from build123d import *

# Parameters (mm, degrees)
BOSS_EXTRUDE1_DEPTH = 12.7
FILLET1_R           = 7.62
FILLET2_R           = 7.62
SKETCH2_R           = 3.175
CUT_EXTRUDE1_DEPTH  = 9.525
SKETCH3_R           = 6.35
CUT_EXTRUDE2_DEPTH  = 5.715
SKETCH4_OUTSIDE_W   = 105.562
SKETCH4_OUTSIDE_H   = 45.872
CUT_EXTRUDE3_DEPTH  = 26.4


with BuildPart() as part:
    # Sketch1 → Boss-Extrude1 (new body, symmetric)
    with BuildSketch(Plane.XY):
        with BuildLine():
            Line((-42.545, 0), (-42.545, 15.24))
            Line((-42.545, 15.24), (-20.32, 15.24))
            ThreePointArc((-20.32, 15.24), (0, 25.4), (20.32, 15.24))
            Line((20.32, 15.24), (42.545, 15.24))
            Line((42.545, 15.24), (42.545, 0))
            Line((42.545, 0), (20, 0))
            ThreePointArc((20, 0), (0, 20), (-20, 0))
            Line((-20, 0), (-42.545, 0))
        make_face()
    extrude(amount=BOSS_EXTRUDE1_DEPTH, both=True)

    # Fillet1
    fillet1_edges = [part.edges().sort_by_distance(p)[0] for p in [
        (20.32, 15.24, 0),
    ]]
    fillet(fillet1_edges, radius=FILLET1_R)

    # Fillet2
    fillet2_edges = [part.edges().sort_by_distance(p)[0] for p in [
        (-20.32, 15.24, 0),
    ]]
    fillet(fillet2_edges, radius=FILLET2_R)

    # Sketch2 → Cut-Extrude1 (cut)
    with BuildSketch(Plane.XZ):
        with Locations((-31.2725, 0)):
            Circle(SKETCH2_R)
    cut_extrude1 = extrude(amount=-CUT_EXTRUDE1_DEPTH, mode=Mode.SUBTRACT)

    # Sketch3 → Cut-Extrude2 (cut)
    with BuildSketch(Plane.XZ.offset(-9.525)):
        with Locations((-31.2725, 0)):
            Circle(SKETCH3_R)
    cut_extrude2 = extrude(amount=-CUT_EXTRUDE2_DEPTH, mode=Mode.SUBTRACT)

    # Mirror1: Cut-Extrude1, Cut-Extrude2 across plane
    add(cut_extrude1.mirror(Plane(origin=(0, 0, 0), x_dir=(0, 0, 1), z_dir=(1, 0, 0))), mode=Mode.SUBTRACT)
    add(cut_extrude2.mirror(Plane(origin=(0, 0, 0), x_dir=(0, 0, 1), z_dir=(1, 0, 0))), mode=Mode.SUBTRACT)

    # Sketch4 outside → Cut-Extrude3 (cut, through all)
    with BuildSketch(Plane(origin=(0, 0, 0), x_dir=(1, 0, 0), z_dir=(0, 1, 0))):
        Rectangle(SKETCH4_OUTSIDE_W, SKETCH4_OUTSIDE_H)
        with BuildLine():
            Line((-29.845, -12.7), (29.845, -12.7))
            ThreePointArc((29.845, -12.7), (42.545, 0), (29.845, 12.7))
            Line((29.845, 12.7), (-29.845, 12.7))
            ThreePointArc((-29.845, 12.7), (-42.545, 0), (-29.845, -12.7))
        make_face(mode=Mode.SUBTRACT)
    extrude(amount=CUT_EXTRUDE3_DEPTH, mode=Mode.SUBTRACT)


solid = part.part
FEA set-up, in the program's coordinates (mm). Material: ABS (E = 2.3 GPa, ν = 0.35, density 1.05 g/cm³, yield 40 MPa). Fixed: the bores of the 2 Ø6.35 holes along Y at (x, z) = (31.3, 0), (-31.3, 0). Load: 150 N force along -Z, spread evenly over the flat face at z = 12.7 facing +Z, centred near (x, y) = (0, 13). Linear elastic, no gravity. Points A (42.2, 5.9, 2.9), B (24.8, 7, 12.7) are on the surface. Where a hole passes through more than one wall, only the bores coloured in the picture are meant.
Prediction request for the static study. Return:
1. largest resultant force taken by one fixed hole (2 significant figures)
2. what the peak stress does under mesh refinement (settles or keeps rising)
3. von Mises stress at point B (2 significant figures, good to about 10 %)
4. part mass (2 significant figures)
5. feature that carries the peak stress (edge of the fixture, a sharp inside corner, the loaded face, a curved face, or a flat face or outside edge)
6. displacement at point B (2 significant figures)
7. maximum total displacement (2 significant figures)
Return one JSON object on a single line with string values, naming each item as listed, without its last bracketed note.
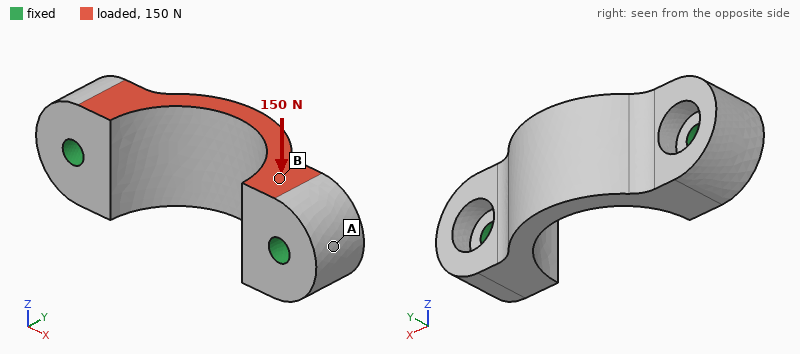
{"largest resultant force taken by one fixed hole": "75 N", "what the peak stress does under mesh refinement": "keeps rising", "von Mises stress at point B": "0.62 MPa", "part mass": "21 g", "feature that carries the peak stress": "edge of the fixture", "displacement at point B": "15 µm", "maximum total displacement": "48 µm"}
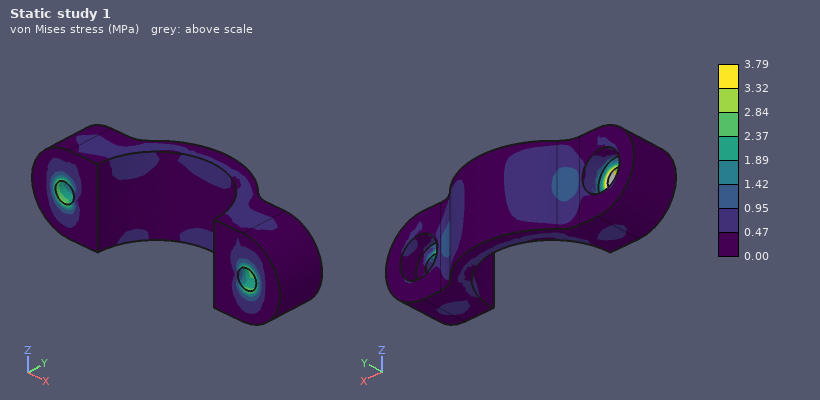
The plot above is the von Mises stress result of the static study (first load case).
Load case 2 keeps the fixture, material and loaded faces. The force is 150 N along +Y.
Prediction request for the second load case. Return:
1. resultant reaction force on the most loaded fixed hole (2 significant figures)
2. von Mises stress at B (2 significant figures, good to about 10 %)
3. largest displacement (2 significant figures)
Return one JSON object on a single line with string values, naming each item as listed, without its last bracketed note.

{"resultant reaction force on the most loaded fixed hole": "82 N", "von Mises stress at B": "0.94 MPa", "largest displacement": "57 µm"}
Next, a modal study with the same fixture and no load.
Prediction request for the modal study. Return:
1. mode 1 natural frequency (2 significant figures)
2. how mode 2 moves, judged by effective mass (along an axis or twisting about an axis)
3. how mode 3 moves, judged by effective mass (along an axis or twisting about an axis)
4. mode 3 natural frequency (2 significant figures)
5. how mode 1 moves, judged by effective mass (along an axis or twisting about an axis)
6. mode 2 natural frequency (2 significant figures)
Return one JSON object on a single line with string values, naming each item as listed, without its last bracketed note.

{"mode 1 natural frequency": "2900 Hz", "how mode 2 moves, judged by effective mass": "along X", "how mode 3 moves, judged by effective mass": "along Y", "mode 3 natural frequency": "5900 Hz", "how mode 1 moves, judged by effective mass": "along Z", "mode 2 natural frequency": "4700 Hz"}
